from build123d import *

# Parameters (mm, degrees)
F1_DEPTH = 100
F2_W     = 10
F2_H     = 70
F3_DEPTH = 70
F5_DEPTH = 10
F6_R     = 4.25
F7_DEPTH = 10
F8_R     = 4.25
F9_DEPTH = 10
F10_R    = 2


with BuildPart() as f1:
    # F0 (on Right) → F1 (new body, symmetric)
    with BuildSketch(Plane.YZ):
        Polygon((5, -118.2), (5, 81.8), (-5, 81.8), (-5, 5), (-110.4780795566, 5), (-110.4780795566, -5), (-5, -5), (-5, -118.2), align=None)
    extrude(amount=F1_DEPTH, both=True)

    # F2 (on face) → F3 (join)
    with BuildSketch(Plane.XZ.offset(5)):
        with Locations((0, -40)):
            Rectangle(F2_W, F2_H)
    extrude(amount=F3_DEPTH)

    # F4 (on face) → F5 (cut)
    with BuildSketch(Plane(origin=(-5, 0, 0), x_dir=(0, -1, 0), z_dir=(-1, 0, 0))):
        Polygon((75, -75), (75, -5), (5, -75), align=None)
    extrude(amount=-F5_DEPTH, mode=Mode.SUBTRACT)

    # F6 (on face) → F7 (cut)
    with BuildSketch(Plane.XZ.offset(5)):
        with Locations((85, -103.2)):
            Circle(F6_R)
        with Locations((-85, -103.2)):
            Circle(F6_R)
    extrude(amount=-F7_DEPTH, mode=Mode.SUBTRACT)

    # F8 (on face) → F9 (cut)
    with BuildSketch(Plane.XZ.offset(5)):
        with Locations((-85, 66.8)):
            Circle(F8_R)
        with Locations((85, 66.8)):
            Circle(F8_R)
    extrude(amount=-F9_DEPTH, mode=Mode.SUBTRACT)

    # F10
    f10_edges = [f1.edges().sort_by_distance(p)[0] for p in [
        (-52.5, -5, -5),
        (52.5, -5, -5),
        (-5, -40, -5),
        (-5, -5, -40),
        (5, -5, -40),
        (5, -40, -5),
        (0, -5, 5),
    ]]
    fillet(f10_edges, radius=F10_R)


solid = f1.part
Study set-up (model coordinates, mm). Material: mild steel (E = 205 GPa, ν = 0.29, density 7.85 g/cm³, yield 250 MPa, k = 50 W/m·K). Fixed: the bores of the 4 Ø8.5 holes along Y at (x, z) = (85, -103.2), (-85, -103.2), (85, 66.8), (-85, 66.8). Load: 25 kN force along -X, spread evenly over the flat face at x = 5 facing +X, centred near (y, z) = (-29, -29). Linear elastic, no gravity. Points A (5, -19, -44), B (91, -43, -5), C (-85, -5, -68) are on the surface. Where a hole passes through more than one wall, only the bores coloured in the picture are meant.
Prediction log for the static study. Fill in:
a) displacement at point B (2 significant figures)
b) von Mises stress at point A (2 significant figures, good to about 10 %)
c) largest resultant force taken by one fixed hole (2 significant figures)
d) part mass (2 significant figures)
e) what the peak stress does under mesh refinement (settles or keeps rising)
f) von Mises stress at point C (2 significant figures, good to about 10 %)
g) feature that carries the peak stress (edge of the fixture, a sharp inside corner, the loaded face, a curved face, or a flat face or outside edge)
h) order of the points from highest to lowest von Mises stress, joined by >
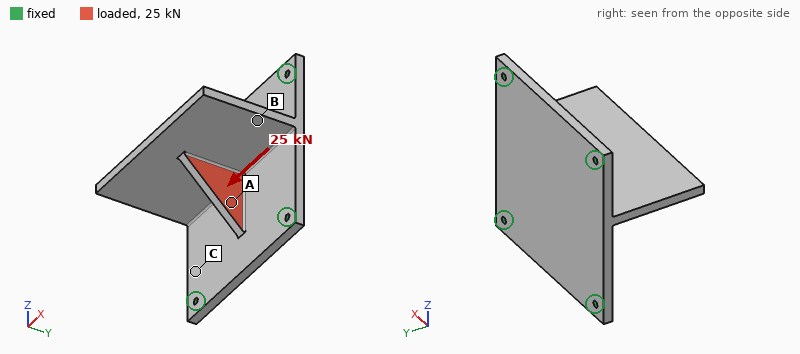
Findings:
0.10 mm
60 MPa
7.6 kN
5.0 kg
keeps rising
25 MPa
edge of the fixture
A > C > B
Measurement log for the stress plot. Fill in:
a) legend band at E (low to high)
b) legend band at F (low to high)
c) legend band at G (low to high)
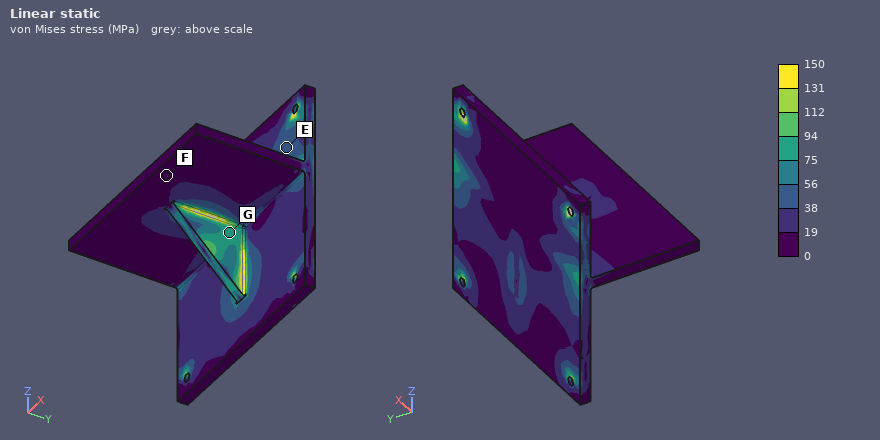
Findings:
38 to 56 MPa
0 to 19 MPa
75 to 94 MPa
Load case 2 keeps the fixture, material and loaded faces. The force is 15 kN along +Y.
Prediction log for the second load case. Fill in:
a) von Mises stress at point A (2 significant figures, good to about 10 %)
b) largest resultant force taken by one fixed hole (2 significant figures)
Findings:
32 MPa
4.3 kN
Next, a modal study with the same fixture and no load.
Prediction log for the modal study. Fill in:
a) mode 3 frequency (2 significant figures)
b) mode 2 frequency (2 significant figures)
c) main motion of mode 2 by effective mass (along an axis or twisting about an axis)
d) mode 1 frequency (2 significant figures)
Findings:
970 Hz
920 Hz
along Y
890 Hz
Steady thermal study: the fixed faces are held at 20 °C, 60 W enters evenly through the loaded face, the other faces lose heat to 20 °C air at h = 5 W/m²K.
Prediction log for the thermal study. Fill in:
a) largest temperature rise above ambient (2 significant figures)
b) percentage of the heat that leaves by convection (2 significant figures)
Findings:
61 K
25 %
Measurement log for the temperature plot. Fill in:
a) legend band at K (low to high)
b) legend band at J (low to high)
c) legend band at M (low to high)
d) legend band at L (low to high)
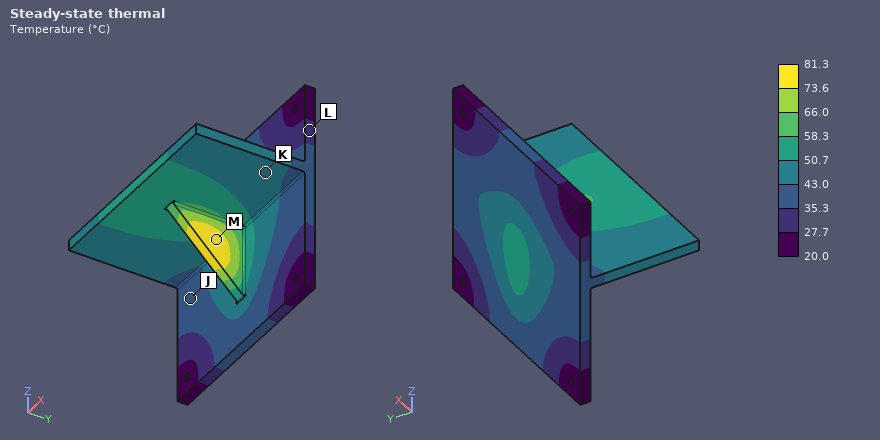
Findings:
43.0 to 50.7 °C
35.3 to 43.0 °C
73.6 to 81.3 °C
27.7 to 35.3 °C
